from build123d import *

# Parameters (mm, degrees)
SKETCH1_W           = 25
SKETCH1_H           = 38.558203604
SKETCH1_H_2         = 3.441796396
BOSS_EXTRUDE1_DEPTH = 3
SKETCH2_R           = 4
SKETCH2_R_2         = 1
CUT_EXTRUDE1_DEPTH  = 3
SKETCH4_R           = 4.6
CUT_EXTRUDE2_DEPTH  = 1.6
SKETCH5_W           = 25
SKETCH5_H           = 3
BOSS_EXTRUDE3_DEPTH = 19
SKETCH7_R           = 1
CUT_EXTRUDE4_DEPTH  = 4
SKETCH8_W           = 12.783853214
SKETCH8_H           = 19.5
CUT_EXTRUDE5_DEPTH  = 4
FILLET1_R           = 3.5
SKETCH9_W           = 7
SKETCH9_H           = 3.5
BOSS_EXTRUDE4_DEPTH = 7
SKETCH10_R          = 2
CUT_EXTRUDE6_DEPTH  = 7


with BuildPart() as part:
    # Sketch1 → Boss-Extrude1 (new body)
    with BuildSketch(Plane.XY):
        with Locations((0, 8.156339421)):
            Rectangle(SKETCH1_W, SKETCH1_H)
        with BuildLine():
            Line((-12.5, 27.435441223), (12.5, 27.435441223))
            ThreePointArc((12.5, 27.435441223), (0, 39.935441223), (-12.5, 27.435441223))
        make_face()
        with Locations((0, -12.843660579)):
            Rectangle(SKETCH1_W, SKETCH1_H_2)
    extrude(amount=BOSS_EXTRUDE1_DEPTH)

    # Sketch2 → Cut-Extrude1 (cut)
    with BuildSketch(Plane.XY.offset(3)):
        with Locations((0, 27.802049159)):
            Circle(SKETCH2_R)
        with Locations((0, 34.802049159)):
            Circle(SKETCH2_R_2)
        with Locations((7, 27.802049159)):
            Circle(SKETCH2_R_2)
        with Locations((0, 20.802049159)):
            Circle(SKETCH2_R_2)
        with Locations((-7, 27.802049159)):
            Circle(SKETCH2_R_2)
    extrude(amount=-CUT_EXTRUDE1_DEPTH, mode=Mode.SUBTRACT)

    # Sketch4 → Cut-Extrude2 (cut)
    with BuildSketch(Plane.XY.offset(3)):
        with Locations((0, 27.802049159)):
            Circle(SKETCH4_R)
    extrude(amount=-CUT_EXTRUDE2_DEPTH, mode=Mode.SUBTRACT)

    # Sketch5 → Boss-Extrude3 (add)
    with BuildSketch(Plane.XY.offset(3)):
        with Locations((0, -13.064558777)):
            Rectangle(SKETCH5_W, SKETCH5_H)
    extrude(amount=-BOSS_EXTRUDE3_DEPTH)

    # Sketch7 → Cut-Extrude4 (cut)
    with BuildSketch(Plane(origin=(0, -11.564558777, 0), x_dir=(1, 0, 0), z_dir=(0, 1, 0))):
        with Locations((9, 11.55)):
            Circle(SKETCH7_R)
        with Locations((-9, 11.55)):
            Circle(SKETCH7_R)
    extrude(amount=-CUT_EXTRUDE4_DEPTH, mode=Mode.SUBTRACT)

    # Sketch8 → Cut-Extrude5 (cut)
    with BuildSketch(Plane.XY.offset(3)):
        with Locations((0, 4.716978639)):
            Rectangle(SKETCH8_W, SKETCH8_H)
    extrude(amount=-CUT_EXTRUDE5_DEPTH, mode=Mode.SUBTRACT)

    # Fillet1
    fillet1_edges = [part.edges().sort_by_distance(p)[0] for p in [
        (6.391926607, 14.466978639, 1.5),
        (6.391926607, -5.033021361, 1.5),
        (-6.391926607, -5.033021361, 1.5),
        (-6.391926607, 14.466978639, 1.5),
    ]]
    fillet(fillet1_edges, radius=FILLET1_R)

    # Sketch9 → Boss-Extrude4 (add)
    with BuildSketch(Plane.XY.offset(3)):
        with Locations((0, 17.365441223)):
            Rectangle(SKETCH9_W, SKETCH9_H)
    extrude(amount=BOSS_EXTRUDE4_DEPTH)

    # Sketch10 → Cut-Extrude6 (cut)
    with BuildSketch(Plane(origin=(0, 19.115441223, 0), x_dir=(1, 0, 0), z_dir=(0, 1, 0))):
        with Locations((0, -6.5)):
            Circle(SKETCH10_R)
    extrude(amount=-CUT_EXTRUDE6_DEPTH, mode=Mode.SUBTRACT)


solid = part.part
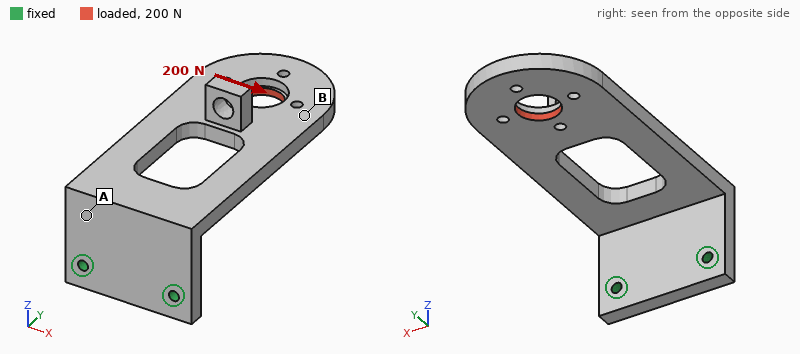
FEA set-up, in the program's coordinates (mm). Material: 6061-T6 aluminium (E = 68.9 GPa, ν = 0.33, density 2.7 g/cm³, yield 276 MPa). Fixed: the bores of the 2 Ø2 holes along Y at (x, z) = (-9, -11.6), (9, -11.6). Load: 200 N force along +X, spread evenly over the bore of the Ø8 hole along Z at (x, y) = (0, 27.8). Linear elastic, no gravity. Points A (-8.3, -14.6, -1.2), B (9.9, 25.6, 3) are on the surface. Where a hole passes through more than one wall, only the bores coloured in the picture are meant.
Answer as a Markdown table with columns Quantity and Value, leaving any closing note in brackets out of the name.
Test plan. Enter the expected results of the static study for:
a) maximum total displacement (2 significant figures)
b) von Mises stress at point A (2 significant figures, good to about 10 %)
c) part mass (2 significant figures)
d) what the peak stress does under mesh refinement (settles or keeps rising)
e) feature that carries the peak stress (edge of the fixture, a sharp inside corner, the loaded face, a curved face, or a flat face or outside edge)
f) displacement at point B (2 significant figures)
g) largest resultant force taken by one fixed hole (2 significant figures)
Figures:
| Quantity | Value |
|---|---|
| maximum total displacement | 0.50 mm |
| von Mises stress at point A | 97 MPa |
| part mass | 12 g |
| what the peak stress does under mesh refinement | keeps rising |
| feature that carries the peak stress | edge of the fixture |
| displacement at point B | 0.37 mm |
| largest resultant force taken by one fixed hole | 460 N |
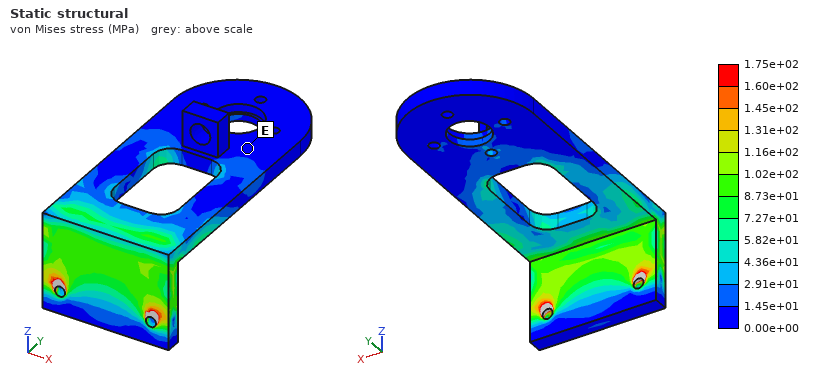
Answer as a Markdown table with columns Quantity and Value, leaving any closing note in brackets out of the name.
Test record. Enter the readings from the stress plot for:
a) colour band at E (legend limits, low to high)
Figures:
| Quantity | Value |
|---|---|
| colour band at E | 0.00e+00 to 1.45e+01 MPa |
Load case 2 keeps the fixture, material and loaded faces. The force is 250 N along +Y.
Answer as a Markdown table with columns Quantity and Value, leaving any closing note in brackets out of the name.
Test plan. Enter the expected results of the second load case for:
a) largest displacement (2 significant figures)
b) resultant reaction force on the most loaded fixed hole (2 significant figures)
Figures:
| Quantity | Value |
|---|---|
| largest displacement | 0.20 mm |
| resultant reaction force on the most loaded fixed hole | 130 N |
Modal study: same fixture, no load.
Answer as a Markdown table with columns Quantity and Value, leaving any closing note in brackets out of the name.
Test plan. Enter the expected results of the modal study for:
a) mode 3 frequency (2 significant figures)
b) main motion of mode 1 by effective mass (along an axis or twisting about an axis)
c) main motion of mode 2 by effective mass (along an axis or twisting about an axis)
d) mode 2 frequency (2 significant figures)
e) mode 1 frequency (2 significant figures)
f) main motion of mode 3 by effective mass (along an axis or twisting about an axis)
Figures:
| Quantity | Value |
|---|---|
| mode 3 frequency | 3300 Hz |
| main motion of mode 1 by effective mass | along Z |
| main motion of mode 2 by effective mass | along X |
| mode 2 frequency | 1700 Hz |
| mode 1 frequency | 640 Hz |
| main motion of mode 3 by effective mass | twisting about Y |
